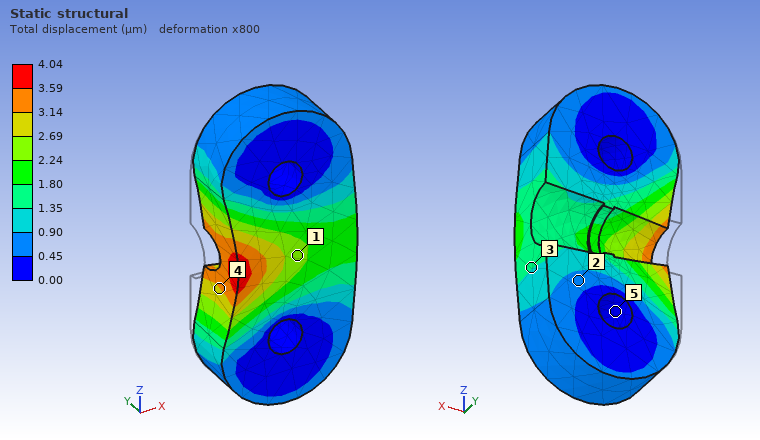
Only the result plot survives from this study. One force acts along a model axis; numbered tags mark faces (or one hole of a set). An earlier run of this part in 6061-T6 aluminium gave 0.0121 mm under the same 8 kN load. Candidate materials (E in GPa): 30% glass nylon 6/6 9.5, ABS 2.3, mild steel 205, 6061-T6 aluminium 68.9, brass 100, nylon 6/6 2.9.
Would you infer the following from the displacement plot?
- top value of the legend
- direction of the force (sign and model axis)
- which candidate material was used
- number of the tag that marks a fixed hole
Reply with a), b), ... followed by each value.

a) 4.04 µm
b) +X
c) mild steel
d) 5
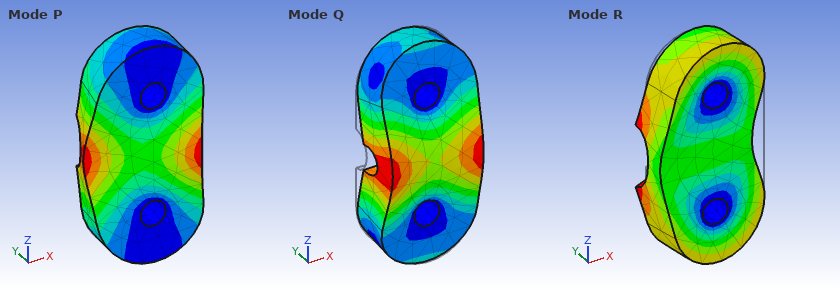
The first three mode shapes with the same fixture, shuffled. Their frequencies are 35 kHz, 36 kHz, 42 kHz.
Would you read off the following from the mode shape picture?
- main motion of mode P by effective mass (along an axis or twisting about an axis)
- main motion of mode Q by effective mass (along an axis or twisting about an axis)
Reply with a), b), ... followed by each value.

a) twisting about Z
b) along Y
